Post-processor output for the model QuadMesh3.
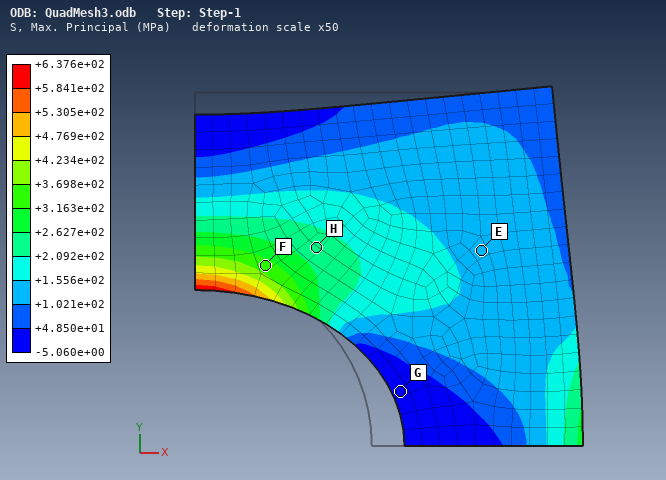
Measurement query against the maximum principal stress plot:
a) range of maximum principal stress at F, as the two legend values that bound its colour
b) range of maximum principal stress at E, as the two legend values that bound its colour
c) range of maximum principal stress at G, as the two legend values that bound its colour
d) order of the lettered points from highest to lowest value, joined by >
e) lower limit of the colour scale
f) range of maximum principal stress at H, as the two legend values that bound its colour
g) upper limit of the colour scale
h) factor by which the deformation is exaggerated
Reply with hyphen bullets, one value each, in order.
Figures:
- +3.163e+02 to +3.698e+02 MPa
- +1.021e+02 to +1.556e+02 MPa
- -5.060e+00 to +4.850e+01 MPa
- F > H > E > G
- -5.060e+00 MPa
- +2.092e+02 to +2.627e+02 MPa
- +6.376e+02 MPa
- 50
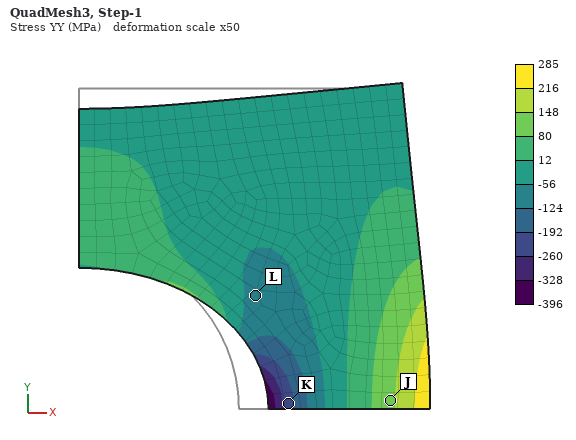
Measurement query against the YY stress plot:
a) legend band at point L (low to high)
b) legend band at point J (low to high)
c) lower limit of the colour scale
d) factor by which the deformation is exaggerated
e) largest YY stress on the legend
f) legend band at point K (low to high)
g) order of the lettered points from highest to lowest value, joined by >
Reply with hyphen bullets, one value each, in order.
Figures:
- -124 to -56 MPa
- 80 to 148 MPa
- -396 MPa
- 50
- 285 MPa
- -260 to -192 MPa
- J > L > K
